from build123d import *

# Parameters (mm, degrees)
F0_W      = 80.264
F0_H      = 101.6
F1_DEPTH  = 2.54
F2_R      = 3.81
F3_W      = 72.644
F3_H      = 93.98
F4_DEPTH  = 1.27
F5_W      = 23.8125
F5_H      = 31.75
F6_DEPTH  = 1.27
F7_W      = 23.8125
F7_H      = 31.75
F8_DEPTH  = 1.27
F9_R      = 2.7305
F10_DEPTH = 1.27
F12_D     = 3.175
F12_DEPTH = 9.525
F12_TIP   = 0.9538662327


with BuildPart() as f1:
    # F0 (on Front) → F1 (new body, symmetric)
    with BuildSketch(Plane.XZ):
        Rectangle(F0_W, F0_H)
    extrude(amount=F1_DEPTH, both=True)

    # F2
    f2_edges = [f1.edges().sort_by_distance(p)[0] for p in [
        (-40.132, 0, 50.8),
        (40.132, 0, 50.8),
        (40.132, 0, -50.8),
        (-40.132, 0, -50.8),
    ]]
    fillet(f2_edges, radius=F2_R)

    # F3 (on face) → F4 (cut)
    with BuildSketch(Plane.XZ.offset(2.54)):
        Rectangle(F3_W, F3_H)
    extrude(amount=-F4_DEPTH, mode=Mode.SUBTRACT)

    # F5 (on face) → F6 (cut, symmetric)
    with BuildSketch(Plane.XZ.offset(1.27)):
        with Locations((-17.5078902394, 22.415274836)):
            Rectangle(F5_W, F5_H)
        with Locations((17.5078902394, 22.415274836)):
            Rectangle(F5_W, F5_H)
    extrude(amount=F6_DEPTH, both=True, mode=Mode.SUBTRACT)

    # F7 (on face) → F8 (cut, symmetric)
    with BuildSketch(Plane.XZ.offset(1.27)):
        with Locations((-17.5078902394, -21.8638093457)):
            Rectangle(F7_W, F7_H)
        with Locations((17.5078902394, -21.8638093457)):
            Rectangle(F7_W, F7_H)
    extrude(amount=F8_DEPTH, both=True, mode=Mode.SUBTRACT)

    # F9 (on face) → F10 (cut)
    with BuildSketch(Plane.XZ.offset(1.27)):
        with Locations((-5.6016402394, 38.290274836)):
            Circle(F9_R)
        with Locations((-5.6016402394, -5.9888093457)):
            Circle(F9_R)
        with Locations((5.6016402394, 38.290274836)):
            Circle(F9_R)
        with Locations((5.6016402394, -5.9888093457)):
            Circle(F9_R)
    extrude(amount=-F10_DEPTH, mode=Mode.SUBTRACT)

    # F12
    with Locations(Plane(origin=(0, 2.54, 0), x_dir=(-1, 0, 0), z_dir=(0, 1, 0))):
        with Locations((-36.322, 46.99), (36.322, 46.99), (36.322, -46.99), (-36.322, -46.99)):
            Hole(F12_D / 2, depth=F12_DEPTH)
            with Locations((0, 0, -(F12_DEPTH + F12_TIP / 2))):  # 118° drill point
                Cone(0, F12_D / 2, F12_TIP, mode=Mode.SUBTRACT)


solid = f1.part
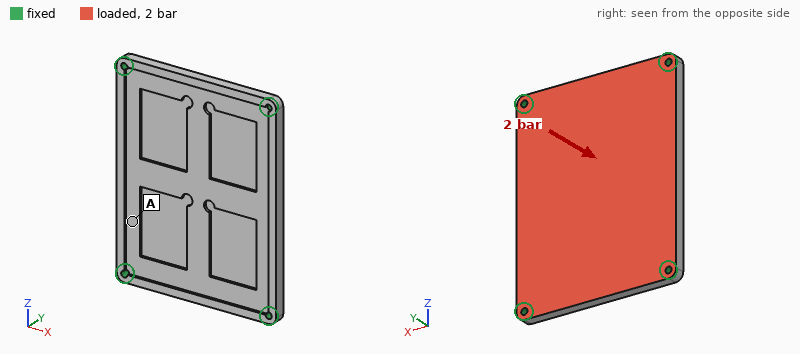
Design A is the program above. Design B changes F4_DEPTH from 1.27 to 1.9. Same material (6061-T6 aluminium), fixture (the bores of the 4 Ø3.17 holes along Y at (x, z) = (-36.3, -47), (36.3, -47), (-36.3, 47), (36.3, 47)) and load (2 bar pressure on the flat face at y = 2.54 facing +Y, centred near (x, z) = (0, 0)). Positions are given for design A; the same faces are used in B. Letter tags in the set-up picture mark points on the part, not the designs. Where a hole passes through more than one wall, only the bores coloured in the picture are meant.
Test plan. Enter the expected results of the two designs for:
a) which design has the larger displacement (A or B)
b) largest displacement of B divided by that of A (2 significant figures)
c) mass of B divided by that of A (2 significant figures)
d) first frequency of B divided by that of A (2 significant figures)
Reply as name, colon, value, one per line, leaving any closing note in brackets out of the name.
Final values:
which design has the larger displacement: B
largest displacement of B divided by that of A: 1.3
mass of B divided by that of A: 0.92
first frequency of B divided by that of A: 0.94
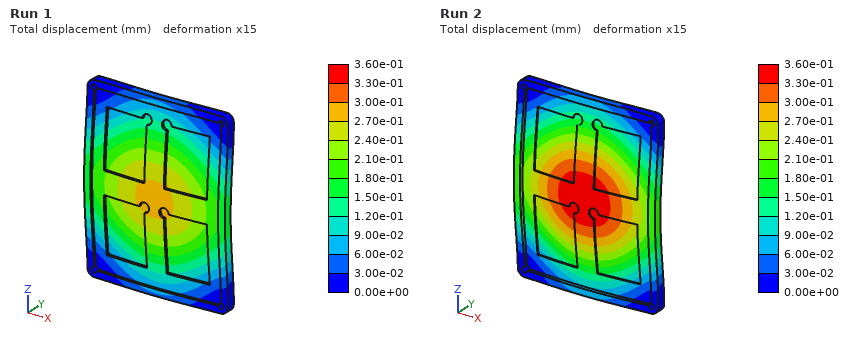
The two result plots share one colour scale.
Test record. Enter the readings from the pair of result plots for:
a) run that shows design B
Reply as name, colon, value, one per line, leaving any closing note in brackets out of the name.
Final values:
run that shows design B: Run 2
